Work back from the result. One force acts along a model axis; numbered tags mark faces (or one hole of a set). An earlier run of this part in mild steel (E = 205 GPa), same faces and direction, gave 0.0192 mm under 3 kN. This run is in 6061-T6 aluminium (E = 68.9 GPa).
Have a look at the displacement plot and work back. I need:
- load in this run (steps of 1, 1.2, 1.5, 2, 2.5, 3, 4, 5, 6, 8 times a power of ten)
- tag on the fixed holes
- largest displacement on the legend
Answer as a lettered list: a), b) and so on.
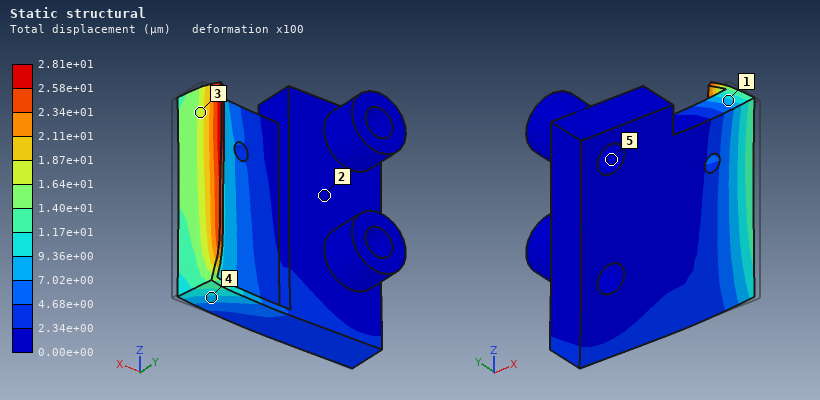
a) 1.5 kN
b) 5
c) 2.81e+01 µm
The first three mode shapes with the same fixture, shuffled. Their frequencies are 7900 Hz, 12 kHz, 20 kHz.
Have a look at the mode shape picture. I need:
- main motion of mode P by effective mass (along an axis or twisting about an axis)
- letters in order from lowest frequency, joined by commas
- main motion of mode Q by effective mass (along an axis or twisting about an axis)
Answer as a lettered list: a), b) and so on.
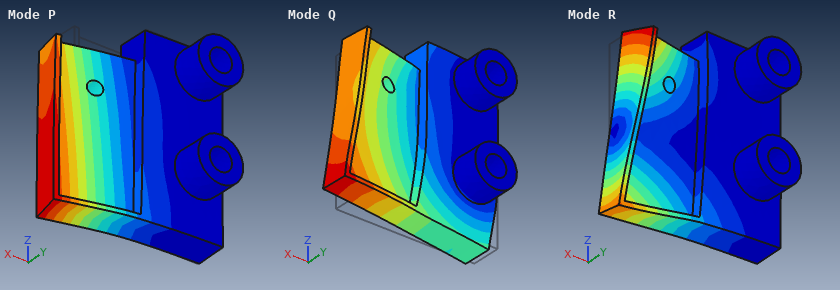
a) along Y
b) P, R, Q
c) along Z
